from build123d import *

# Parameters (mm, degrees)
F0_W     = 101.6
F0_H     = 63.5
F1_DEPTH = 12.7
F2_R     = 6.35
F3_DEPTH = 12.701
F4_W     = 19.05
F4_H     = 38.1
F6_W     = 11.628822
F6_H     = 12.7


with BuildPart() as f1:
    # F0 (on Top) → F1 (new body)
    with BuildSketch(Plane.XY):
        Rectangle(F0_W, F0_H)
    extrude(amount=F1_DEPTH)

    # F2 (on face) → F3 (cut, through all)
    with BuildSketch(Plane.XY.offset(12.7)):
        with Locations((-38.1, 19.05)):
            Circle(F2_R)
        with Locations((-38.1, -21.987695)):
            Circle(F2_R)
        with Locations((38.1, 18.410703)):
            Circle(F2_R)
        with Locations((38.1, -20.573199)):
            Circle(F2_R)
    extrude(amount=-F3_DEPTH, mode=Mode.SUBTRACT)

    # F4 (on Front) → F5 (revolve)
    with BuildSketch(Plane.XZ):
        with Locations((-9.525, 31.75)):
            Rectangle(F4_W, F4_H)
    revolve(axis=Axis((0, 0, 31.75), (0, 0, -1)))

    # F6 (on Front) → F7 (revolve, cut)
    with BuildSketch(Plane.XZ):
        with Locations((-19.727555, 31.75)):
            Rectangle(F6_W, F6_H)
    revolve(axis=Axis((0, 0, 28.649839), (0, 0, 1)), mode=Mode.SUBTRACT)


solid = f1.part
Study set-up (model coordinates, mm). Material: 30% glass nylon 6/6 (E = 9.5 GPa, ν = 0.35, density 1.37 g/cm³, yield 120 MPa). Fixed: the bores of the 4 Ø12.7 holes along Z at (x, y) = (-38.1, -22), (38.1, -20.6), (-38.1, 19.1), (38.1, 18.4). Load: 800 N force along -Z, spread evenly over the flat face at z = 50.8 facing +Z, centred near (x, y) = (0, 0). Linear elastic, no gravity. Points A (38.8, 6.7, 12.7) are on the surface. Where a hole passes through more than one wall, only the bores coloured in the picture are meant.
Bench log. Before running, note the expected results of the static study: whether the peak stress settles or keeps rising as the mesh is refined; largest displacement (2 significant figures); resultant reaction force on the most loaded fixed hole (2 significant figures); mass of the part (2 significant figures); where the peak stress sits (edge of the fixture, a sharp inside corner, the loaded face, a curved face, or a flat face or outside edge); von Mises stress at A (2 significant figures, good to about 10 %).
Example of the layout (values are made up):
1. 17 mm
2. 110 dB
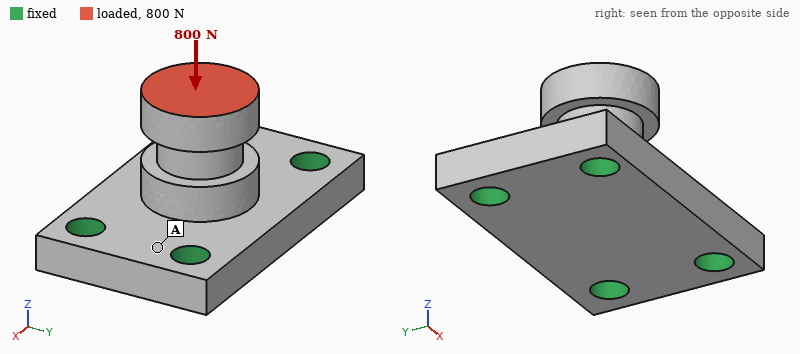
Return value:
1. keeps rising
2. 15 µm
3. 220 N
4. 150 g
5. edge of the fixture
6. 0.88 MPa
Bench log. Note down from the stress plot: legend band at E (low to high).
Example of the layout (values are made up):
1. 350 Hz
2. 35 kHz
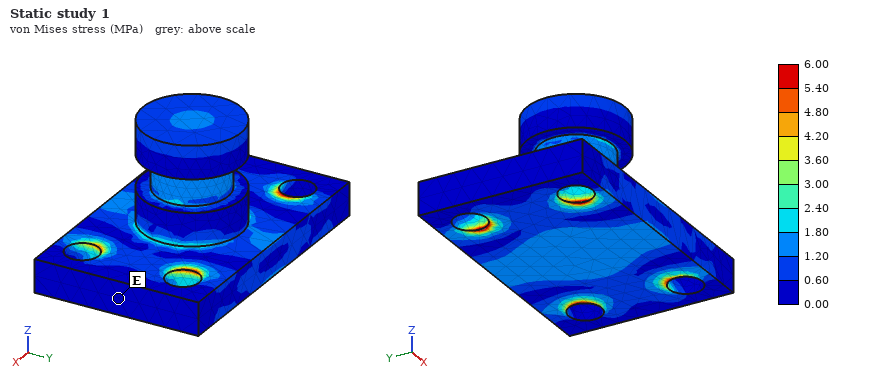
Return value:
1. 0.00 to 0.60 MPa
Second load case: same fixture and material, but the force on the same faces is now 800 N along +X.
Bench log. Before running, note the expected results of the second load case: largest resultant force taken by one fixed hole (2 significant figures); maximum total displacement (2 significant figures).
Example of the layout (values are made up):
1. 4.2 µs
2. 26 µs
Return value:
1. 410 N
2. 85 µm
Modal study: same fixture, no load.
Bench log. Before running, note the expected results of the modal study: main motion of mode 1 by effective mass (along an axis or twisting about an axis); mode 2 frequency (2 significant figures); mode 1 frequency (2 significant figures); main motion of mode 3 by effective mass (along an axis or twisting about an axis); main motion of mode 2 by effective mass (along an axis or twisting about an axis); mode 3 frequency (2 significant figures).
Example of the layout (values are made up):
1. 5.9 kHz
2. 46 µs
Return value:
1. along Y
2. 3900 Hz
3. 3000 Hz
4. along Z
5. along X
6. 4500 Hz
